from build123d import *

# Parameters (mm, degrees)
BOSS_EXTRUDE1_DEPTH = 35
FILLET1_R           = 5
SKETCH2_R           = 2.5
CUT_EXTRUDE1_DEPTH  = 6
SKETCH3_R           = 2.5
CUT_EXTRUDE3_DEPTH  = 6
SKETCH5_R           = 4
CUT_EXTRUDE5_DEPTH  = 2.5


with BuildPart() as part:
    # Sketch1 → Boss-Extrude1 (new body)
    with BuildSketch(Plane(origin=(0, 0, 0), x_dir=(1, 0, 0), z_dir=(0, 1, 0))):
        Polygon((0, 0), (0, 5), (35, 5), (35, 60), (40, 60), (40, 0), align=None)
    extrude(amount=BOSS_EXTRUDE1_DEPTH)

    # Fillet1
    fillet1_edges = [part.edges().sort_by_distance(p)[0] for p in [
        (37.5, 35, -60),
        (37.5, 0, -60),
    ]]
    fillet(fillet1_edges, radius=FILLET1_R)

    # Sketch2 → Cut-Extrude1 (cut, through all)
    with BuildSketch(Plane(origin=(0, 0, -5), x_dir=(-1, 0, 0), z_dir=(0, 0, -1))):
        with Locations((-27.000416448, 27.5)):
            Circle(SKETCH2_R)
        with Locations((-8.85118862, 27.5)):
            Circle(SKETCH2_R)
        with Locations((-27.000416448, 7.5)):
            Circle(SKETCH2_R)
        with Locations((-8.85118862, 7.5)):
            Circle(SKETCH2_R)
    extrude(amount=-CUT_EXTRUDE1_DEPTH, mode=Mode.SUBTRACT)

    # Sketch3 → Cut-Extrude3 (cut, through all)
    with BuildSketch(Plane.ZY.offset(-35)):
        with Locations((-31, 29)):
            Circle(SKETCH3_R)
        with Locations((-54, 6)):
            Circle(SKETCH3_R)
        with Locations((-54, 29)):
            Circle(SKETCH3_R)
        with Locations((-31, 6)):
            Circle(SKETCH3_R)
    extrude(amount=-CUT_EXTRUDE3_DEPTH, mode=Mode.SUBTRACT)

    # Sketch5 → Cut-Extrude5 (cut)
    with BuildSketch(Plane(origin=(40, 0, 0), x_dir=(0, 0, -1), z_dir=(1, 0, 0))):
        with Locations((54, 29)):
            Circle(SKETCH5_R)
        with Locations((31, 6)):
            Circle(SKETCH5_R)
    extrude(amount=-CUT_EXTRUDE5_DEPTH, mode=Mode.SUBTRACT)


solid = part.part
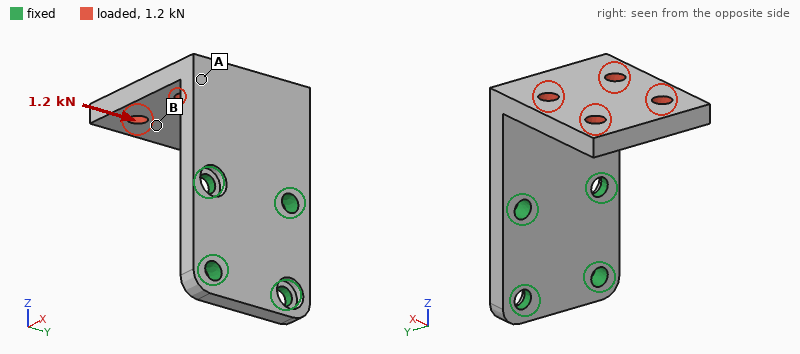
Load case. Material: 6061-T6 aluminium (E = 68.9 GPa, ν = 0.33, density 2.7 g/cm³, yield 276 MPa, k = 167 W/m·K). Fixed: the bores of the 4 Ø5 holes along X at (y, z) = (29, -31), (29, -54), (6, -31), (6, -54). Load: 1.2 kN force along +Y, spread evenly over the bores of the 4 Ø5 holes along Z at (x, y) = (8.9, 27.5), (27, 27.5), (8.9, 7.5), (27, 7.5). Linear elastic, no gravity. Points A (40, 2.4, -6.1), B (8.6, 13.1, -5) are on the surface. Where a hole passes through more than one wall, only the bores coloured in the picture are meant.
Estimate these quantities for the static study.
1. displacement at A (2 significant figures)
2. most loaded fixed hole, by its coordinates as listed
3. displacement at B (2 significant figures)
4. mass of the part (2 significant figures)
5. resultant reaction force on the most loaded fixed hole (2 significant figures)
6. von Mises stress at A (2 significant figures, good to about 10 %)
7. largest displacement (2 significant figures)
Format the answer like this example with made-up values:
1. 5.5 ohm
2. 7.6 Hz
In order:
1. 0.19 mm
2. (29, -31)
3. 0.38 mm
4. 42 g
5. 1.6 kN
6. 80 MPa
7. 0.54 mm
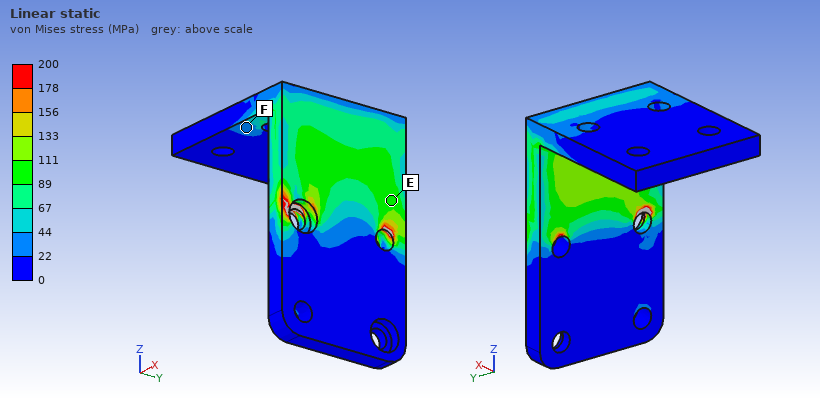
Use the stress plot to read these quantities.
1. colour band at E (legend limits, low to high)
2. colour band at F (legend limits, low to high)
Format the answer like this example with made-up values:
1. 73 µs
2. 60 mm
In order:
1. 89 to 111 MPa
2. 22 to 44 MPa
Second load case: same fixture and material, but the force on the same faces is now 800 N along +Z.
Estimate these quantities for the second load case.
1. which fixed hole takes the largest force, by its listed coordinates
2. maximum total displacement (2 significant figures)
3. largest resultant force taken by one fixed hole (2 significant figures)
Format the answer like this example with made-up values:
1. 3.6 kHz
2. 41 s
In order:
1. (6, -31)
2. 0.90 mm
3. 740 N
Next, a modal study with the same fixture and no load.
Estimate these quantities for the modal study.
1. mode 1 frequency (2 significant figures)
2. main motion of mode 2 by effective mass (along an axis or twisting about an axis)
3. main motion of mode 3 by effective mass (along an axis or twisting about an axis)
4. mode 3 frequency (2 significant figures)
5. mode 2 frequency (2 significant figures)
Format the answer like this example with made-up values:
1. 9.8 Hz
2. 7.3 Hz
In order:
1. 1300 Hz
2. along Y
3. along X
4. 3500 Hz
5. 2200 Hz
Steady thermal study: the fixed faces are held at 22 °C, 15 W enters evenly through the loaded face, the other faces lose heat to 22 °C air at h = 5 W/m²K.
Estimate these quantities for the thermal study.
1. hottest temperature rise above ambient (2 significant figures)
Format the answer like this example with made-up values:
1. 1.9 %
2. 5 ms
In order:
1. 25 K
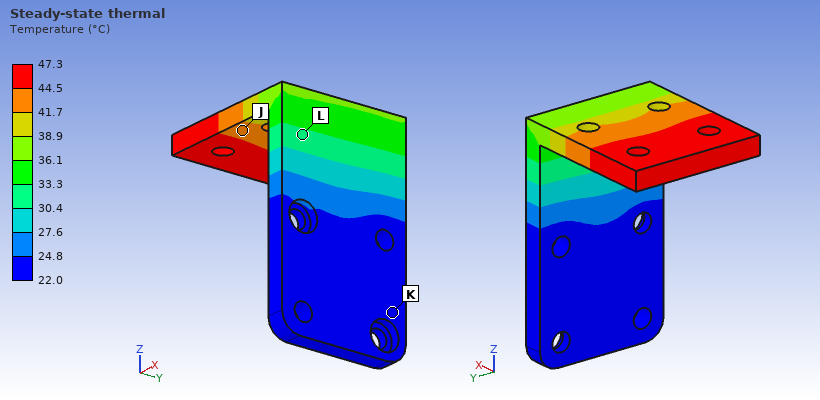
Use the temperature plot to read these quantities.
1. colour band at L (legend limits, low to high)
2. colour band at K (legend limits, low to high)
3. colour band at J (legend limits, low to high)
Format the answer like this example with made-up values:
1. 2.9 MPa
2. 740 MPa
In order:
1. 30.4 to 33.3 °C
2. 22.0 to 24.8 °C
3. 41.7 to 44.5 °C
